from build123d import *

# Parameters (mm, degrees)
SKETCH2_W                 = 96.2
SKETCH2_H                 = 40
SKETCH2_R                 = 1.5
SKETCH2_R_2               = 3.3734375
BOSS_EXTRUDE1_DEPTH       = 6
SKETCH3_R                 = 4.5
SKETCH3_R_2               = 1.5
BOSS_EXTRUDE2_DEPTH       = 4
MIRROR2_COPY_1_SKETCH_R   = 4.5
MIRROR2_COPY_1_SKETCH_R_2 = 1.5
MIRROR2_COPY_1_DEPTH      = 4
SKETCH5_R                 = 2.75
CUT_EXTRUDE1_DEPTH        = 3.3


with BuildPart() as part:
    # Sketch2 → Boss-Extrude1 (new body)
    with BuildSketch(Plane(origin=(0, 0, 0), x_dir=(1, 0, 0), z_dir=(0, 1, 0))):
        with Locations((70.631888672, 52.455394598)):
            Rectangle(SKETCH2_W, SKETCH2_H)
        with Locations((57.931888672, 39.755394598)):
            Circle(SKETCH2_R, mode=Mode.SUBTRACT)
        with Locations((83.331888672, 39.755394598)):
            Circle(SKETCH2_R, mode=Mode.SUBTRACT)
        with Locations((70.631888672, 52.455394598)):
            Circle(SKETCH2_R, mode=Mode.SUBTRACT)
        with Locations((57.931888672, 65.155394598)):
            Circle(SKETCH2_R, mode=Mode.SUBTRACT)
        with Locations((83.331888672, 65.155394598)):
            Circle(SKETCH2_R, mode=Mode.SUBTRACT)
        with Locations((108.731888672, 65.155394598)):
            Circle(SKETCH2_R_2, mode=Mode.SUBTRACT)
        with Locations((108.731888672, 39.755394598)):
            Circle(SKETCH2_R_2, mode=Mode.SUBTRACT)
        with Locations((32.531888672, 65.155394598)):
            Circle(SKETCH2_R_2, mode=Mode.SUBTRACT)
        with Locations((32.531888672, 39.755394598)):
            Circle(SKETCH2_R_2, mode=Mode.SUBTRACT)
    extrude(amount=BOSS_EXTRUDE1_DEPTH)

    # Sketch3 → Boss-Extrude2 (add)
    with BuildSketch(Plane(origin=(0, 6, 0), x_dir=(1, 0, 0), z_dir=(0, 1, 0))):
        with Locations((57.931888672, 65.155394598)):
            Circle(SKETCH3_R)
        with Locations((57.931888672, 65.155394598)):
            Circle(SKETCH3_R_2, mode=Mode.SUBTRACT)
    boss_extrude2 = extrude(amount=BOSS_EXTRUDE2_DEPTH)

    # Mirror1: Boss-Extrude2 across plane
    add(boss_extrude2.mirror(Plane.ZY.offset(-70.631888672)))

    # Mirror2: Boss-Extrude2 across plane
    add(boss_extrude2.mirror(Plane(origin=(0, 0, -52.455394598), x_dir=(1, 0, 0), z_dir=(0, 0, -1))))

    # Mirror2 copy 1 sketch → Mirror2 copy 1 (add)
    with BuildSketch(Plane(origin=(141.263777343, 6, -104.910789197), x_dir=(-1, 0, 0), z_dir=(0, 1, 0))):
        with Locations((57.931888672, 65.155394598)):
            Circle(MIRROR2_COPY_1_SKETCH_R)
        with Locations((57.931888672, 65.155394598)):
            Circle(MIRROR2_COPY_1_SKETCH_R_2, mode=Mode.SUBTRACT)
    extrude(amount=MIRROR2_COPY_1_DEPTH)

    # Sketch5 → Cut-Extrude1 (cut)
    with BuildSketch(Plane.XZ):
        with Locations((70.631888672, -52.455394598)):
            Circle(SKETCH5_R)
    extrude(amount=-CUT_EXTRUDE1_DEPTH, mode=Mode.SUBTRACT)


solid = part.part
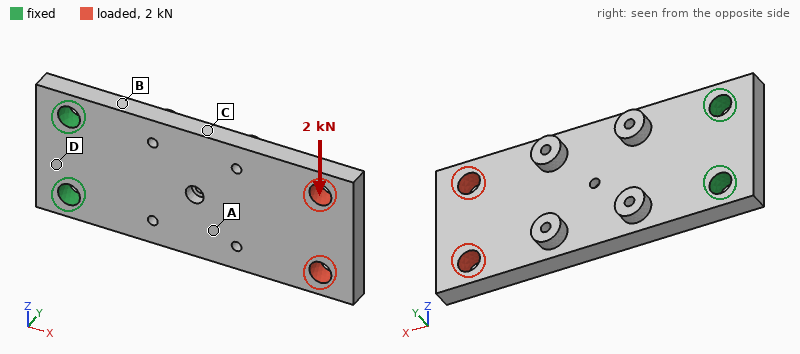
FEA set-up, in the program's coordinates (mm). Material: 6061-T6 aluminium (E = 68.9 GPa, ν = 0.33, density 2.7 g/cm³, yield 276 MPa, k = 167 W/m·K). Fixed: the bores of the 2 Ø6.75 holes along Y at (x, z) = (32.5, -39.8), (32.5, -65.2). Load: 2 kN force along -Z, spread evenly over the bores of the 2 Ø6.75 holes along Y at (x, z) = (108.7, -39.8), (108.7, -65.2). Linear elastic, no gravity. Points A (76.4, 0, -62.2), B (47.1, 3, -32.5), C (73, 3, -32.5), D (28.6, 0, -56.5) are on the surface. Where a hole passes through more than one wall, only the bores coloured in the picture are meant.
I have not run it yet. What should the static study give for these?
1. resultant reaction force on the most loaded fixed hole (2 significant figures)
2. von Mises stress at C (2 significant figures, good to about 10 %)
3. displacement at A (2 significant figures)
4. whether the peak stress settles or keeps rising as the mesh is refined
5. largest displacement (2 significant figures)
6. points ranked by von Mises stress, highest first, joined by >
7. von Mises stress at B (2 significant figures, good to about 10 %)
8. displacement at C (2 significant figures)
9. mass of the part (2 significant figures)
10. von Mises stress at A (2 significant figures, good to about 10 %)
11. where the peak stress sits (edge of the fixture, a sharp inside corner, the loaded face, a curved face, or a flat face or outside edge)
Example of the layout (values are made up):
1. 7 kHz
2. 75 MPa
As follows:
1. 5.4 kN
2. 45 MPa
3. 0.073 mm
4. keeps rising
5. 0.20 mm
6. B > C > A > D
7. 74 MPa
8. 0.075 mm
9. 62 g
10. 27 MPa
11. edge of the fixture
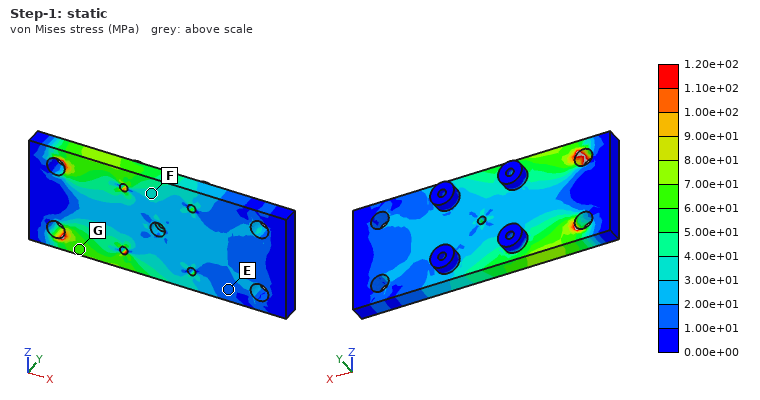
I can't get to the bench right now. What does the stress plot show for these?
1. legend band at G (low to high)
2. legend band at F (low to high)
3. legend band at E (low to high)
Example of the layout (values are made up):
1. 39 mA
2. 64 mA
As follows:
1. 6.00e+01 to 7.00e+01 MPa
2. 3.00e+01 to 4.00e+01 MPa
3. 1.00e+01 to 2.00e+01 MPa
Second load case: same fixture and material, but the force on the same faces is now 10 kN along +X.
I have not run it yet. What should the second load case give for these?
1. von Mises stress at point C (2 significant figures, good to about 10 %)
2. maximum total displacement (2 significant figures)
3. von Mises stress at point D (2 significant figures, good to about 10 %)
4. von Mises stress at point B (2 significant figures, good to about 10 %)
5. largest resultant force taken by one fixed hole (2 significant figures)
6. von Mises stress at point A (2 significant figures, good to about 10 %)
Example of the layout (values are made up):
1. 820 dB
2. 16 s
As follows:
1. 42 MPa
2. 66 µm
3. 16 MPa
4. 42 MPa
5. 5.1 kN
6. 45 MPa
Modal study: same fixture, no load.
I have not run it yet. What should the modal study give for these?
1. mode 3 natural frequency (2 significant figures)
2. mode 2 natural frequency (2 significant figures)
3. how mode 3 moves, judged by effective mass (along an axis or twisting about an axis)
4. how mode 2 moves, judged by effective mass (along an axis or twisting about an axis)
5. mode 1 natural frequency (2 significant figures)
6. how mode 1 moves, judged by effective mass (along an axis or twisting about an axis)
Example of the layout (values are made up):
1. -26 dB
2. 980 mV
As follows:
1. 3900 Hz
2. 3000 Hz
3. along Z
4. twisting about X
5. 710 Hz
6. along Y
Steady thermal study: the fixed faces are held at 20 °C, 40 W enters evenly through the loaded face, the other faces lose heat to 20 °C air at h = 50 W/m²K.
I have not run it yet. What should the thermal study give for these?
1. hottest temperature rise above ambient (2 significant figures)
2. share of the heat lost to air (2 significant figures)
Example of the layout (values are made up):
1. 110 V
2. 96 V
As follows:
1. 61 K
2. 34 %
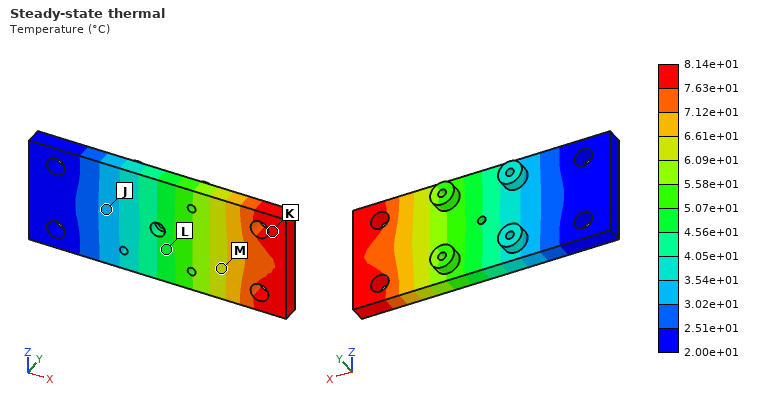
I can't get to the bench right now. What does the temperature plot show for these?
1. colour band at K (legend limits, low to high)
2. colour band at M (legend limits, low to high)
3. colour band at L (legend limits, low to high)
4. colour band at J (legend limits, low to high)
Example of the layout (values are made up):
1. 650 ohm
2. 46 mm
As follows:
1. 7.63e+01 to 8.14e+01 °C
2. 6.09e+01 to 6.61e+01 °C
3. 4.56e+01 to 5.07e+01 °C
4. 3.02e+01 to 3.54e+01 °C
